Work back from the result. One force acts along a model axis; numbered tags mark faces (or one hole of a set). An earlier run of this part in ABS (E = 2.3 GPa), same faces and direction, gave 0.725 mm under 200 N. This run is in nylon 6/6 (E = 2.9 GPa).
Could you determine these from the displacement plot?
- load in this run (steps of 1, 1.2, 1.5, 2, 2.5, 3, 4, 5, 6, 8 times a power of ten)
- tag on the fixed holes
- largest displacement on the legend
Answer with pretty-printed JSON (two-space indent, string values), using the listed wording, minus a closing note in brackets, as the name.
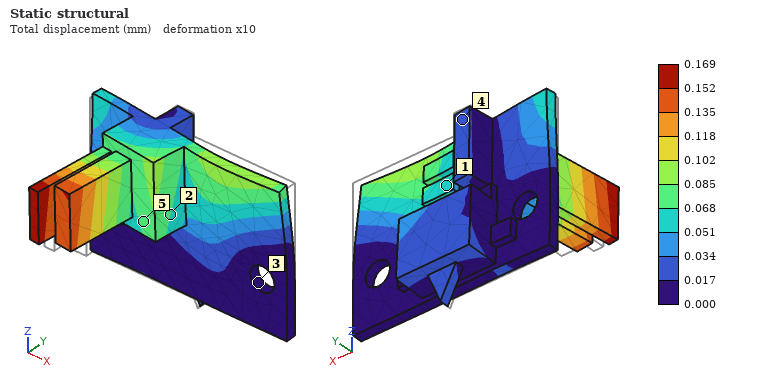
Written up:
{
  "load in this run": "60 N",
  "tag on the fixed holes": "3",
  "largest displacement on the legend": "0.169 mm"
}
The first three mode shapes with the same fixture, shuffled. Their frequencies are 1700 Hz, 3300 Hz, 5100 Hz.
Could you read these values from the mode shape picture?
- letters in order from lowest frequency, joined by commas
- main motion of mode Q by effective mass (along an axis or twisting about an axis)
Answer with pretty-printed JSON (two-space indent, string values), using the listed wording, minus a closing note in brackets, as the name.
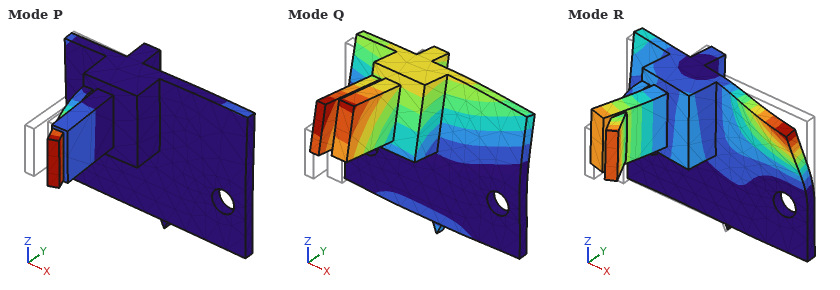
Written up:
{
  "letters in order from lowest frequency, joined by commas": "Q, P, R",
  "main motion of mode Q by effective mass": "along Y"
}
